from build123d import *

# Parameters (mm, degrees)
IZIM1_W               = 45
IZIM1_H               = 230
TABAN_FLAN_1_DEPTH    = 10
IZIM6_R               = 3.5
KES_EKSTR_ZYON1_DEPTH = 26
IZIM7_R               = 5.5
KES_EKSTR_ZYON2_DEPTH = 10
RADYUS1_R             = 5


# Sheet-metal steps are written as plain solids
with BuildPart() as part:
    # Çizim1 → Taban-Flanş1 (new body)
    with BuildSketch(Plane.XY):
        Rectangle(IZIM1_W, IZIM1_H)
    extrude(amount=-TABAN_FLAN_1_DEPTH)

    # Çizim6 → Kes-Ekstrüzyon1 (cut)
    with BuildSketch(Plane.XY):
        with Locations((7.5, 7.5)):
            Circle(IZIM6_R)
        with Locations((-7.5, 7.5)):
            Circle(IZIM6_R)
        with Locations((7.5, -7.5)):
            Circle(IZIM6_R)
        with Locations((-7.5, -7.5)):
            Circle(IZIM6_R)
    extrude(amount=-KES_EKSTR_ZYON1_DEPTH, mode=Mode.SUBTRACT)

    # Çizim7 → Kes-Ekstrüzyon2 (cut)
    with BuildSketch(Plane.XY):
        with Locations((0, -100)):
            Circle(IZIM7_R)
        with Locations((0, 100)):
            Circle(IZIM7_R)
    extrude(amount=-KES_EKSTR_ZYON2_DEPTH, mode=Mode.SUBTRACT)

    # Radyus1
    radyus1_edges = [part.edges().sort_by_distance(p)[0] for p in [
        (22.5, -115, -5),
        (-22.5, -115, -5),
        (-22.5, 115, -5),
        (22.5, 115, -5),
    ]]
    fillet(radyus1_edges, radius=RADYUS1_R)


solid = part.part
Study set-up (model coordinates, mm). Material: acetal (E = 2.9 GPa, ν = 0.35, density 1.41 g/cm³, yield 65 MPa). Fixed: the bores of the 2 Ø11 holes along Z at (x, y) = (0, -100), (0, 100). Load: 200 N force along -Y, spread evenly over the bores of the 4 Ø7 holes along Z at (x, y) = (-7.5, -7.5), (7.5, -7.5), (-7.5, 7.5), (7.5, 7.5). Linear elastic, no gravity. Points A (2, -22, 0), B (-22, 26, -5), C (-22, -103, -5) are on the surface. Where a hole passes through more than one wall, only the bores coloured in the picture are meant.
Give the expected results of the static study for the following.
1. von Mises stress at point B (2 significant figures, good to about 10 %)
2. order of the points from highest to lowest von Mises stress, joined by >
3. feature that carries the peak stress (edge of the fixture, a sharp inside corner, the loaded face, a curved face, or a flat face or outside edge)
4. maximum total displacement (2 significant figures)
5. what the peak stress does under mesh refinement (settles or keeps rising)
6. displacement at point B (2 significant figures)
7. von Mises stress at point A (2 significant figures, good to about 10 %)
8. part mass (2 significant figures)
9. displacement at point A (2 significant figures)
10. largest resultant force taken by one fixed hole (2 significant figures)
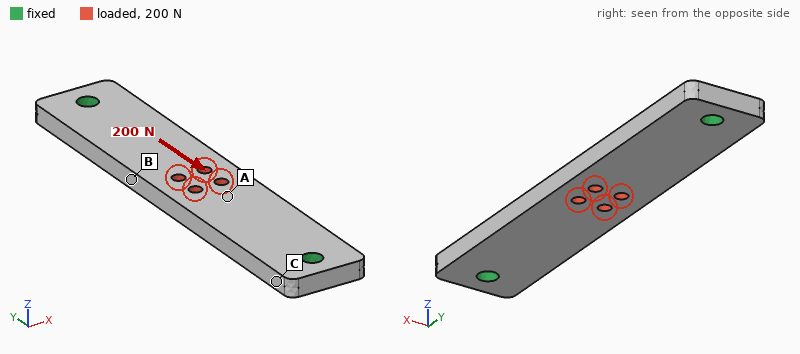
0.19 MPa
A > B > C
edge of the fixture
9.1 µm
keeps rising
6.3 µm
0.30 MPa
140 g
6.9 µm
100 N
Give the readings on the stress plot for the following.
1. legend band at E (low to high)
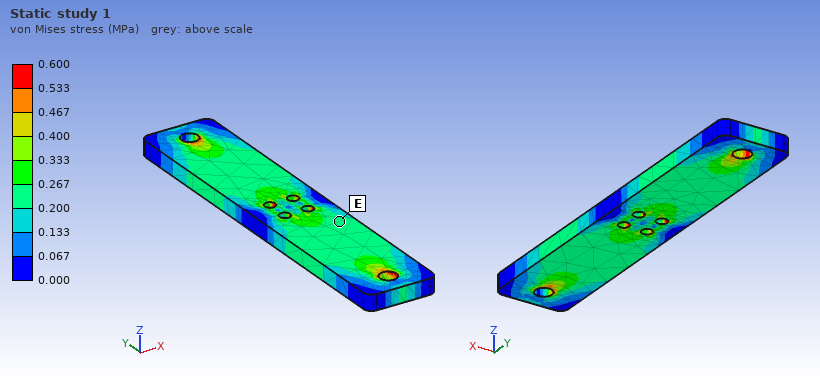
0.200 to 0.267 MPa
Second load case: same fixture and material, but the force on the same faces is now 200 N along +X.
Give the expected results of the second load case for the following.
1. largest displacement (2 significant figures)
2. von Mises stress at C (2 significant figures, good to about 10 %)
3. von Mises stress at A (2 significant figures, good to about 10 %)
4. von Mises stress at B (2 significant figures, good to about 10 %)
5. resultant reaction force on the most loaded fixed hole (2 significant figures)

97 µm
0.34 MPa
0.45 MPa
1.2 MPa
100 N
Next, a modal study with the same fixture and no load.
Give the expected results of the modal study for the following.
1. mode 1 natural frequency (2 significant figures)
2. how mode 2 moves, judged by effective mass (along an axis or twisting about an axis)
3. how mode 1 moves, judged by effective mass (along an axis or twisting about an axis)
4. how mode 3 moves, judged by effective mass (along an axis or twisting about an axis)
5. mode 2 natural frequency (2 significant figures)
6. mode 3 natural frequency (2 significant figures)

370 Hz
twisting about Y
along Z
along X
920 Hz
980 Hz
